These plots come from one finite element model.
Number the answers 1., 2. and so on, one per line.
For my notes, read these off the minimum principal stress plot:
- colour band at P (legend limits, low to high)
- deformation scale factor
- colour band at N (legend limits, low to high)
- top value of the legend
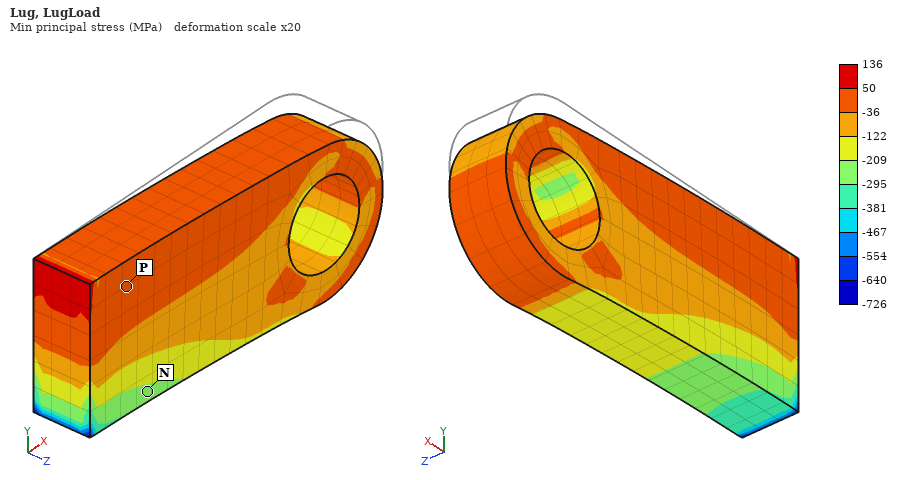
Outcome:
1. -36 to 50 MPa
2. 20
3. -295 to -209 MPa
4. 136 MPa
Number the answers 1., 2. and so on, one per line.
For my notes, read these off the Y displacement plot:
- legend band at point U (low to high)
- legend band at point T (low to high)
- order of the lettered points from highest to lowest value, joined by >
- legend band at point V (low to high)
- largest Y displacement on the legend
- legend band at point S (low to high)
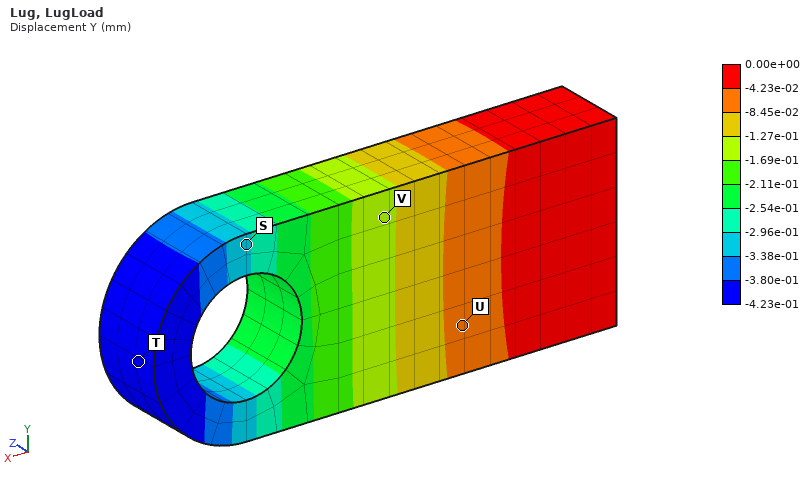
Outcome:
1. -8.45e-02 to -4.23e-02 mm
2. -4.23e-01 to -3.80e-01 mm
3. U > V > S > T
4. -1.69e-01 to -1.27e-01 mm
5. 0.00e+00 mm
6. -3.38e-01 to -2.96e-01 mm
